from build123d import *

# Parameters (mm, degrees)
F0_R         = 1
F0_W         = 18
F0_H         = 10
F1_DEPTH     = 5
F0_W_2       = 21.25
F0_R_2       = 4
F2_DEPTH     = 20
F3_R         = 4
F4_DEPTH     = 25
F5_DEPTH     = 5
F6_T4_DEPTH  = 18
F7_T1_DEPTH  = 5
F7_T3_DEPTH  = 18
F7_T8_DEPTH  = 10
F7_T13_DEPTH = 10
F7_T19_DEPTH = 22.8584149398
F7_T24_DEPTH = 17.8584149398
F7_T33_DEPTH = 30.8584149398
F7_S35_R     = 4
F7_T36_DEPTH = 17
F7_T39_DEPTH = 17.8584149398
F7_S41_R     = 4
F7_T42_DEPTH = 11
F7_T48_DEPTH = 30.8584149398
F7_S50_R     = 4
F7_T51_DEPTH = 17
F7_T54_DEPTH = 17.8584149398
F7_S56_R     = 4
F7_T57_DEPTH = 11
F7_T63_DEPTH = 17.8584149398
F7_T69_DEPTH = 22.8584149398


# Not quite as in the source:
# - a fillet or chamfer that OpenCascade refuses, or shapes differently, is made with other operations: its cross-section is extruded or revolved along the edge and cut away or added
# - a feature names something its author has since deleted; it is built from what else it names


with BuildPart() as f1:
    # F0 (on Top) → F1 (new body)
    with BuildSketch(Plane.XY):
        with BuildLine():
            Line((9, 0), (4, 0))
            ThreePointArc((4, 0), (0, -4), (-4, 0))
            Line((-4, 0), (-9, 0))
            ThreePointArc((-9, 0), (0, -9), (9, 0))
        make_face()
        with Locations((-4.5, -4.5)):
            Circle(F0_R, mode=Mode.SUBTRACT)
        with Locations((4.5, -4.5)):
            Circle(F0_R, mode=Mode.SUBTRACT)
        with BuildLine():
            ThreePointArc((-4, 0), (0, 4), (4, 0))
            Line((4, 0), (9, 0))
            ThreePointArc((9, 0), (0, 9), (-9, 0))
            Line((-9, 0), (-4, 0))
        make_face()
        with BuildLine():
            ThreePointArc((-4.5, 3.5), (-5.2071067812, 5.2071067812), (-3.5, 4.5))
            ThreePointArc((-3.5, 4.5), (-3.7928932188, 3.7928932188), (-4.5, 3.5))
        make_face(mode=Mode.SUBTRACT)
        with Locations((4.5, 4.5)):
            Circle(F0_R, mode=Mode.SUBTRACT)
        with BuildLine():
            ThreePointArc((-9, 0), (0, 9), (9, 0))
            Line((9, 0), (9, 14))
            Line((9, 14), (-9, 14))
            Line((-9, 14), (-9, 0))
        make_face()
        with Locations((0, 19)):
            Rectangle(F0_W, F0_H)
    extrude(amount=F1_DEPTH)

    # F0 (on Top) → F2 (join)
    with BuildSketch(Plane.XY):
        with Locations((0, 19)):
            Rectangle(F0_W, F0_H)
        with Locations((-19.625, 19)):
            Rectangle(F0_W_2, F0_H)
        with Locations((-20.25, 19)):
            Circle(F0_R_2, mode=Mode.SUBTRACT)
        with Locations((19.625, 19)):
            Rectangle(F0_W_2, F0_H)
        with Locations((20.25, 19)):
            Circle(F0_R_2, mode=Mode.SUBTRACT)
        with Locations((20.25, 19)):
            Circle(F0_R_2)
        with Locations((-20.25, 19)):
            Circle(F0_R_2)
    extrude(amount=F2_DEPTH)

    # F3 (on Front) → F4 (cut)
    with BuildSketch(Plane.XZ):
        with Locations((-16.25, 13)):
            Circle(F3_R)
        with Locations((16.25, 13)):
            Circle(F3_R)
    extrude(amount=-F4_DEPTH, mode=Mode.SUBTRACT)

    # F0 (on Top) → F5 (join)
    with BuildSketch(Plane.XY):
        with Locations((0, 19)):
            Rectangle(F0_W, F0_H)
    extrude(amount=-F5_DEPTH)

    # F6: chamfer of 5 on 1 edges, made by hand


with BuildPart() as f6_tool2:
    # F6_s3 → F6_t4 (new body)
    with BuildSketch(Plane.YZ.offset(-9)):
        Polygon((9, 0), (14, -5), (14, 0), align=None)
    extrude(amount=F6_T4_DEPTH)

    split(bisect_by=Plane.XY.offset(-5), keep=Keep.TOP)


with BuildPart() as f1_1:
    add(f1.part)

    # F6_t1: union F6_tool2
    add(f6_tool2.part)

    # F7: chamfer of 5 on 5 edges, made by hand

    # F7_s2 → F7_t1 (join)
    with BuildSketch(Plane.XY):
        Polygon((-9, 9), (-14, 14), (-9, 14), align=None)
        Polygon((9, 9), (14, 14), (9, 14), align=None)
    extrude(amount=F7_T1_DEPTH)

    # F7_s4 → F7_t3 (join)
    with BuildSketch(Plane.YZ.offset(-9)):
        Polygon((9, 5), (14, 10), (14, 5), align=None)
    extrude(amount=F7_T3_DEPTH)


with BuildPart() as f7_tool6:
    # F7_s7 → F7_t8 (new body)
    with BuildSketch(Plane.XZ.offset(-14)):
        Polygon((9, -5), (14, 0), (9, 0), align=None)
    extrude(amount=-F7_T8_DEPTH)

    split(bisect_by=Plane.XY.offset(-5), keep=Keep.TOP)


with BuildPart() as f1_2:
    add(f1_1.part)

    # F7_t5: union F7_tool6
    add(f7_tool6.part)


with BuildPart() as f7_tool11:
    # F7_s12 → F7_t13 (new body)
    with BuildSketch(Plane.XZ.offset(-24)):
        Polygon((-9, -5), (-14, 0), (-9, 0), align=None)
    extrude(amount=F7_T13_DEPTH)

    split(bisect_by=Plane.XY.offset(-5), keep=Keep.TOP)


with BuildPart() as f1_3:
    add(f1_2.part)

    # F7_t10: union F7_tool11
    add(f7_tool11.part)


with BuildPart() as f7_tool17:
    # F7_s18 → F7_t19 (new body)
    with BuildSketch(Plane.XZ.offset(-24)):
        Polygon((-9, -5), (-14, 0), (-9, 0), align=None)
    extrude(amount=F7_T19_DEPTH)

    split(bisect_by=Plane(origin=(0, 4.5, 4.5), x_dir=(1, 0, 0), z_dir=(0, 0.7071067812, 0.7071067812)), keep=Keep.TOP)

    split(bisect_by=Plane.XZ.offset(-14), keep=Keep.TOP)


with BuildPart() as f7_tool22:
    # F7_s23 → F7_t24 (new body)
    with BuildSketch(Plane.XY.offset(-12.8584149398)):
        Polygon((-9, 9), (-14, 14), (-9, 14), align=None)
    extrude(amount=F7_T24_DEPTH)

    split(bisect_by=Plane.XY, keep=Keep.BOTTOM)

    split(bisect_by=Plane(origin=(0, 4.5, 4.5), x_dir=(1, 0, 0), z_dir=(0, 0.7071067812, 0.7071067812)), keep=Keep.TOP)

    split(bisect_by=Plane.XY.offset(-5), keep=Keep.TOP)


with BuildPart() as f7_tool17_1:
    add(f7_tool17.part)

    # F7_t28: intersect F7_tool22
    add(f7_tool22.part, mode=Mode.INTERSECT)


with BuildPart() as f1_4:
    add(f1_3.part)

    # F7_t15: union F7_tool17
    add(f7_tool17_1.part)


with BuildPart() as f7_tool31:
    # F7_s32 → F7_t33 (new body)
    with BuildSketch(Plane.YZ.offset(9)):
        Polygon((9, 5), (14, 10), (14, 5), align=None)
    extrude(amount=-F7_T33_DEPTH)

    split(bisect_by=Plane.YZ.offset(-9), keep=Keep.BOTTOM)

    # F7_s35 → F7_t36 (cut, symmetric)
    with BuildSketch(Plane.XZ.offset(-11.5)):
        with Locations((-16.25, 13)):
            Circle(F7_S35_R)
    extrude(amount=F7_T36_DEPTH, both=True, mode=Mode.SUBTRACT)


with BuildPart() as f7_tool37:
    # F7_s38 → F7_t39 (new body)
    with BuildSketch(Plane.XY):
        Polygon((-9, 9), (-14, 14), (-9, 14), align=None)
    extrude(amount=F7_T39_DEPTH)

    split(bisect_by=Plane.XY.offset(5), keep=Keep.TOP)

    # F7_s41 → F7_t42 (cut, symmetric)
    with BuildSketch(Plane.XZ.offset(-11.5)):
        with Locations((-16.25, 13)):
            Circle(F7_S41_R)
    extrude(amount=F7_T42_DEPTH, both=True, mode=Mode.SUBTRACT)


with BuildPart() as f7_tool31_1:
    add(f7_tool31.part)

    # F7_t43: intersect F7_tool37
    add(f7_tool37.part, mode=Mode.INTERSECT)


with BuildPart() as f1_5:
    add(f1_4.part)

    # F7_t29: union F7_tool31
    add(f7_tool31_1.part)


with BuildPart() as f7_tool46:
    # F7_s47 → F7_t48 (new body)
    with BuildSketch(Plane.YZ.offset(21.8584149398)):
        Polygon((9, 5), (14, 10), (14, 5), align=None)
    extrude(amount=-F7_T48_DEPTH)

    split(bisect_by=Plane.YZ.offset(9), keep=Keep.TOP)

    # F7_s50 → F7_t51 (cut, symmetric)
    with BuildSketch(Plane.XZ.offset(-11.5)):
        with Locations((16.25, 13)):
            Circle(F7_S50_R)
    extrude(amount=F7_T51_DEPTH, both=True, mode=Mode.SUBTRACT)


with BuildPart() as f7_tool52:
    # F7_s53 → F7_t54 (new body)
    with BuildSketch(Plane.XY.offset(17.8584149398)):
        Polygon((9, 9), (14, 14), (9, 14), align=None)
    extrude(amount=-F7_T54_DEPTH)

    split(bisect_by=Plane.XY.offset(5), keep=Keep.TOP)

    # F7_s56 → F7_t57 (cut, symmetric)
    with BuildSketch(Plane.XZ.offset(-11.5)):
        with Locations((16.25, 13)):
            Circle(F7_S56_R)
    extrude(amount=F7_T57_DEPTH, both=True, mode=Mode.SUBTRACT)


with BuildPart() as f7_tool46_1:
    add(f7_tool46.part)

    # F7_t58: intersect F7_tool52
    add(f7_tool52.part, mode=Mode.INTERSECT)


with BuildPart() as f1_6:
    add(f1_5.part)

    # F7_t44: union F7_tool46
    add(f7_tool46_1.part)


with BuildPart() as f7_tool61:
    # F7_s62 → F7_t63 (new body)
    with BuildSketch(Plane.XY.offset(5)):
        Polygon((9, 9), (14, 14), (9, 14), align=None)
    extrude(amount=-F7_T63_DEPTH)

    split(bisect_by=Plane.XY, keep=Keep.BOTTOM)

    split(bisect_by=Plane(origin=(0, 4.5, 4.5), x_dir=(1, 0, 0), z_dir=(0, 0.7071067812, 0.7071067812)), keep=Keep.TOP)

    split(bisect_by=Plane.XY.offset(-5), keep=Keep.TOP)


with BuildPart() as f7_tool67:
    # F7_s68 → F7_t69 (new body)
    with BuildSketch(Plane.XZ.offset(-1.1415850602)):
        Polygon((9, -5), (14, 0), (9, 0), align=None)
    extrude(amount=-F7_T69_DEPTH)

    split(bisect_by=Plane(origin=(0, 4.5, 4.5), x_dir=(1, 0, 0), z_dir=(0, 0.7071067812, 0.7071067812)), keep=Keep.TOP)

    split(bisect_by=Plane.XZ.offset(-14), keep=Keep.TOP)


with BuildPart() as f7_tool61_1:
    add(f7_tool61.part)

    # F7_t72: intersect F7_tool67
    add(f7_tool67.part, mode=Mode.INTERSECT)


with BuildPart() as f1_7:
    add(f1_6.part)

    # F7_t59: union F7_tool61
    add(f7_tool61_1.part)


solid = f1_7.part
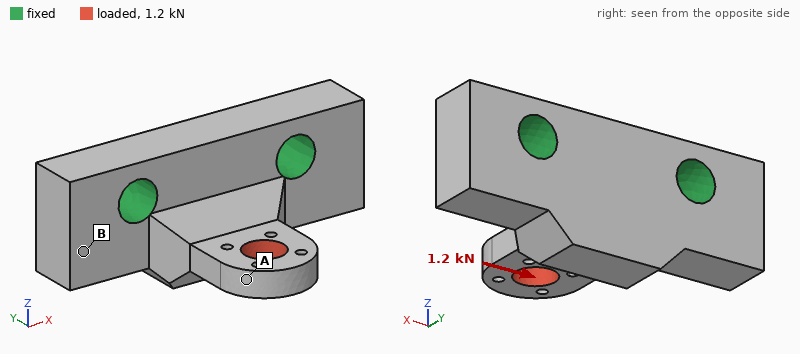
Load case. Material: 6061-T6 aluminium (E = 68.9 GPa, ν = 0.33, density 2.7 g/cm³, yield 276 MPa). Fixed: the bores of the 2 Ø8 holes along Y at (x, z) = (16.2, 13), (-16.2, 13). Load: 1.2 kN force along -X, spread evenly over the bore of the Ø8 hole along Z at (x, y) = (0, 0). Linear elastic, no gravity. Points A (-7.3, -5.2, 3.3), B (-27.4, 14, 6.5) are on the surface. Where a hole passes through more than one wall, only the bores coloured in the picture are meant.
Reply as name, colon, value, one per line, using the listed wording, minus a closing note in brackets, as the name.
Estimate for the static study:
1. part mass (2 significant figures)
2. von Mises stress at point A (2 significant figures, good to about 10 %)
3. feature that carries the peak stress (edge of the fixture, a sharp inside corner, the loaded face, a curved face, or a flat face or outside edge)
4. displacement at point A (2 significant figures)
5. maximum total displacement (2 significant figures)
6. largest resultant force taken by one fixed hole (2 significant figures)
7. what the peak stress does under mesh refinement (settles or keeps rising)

part mass: 39 g
von Mises stress at point A: 19 MPa
feature that carries the peak stress: a sharp inside corner
displacement at point A: 28 µm
maximum total displacement: 30 µm
largest resultant force taken by one fixed hole: 1.0 kN
what the peak stress does under mesh refinement: keeps rising
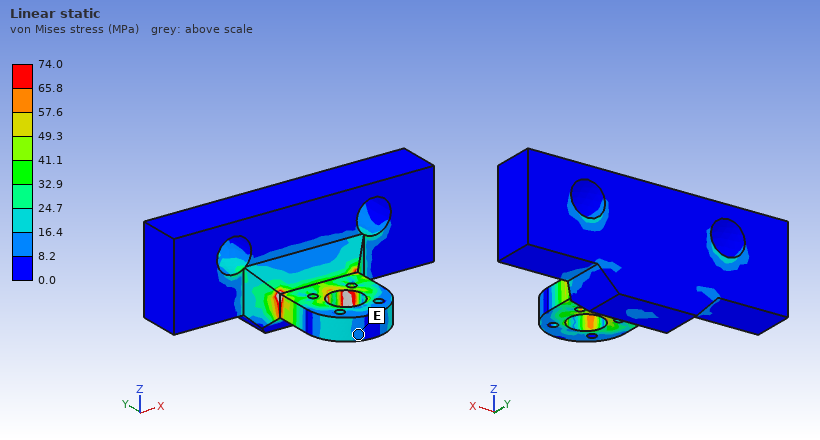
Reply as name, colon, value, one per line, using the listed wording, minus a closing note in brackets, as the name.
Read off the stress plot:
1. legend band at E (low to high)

legend band at E: 8.2 to 16.4 MPa
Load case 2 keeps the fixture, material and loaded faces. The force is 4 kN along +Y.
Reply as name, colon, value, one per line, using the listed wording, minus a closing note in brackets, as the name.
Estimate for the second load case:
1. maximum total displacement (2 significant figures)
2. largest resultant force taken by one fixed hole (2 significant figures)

maximum total displacement: 48 µm
largest resultant force taken by one fixed hole: 2.0 kN
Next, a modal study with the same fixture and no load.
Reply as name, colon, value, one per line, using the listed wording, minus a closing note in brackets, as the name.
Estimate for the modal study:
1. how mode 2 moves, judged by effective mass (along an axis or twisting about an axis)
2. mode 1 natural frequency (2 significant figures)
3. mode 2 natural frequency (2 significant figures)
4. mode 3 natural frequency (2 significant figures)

how mode 2 moves, judged by effective mass: along Y
mode 1 natural frequency: 10 kHz
mode 2 natural frequency: 20 kHz
mode 3 natural frequency: 21 kHz
